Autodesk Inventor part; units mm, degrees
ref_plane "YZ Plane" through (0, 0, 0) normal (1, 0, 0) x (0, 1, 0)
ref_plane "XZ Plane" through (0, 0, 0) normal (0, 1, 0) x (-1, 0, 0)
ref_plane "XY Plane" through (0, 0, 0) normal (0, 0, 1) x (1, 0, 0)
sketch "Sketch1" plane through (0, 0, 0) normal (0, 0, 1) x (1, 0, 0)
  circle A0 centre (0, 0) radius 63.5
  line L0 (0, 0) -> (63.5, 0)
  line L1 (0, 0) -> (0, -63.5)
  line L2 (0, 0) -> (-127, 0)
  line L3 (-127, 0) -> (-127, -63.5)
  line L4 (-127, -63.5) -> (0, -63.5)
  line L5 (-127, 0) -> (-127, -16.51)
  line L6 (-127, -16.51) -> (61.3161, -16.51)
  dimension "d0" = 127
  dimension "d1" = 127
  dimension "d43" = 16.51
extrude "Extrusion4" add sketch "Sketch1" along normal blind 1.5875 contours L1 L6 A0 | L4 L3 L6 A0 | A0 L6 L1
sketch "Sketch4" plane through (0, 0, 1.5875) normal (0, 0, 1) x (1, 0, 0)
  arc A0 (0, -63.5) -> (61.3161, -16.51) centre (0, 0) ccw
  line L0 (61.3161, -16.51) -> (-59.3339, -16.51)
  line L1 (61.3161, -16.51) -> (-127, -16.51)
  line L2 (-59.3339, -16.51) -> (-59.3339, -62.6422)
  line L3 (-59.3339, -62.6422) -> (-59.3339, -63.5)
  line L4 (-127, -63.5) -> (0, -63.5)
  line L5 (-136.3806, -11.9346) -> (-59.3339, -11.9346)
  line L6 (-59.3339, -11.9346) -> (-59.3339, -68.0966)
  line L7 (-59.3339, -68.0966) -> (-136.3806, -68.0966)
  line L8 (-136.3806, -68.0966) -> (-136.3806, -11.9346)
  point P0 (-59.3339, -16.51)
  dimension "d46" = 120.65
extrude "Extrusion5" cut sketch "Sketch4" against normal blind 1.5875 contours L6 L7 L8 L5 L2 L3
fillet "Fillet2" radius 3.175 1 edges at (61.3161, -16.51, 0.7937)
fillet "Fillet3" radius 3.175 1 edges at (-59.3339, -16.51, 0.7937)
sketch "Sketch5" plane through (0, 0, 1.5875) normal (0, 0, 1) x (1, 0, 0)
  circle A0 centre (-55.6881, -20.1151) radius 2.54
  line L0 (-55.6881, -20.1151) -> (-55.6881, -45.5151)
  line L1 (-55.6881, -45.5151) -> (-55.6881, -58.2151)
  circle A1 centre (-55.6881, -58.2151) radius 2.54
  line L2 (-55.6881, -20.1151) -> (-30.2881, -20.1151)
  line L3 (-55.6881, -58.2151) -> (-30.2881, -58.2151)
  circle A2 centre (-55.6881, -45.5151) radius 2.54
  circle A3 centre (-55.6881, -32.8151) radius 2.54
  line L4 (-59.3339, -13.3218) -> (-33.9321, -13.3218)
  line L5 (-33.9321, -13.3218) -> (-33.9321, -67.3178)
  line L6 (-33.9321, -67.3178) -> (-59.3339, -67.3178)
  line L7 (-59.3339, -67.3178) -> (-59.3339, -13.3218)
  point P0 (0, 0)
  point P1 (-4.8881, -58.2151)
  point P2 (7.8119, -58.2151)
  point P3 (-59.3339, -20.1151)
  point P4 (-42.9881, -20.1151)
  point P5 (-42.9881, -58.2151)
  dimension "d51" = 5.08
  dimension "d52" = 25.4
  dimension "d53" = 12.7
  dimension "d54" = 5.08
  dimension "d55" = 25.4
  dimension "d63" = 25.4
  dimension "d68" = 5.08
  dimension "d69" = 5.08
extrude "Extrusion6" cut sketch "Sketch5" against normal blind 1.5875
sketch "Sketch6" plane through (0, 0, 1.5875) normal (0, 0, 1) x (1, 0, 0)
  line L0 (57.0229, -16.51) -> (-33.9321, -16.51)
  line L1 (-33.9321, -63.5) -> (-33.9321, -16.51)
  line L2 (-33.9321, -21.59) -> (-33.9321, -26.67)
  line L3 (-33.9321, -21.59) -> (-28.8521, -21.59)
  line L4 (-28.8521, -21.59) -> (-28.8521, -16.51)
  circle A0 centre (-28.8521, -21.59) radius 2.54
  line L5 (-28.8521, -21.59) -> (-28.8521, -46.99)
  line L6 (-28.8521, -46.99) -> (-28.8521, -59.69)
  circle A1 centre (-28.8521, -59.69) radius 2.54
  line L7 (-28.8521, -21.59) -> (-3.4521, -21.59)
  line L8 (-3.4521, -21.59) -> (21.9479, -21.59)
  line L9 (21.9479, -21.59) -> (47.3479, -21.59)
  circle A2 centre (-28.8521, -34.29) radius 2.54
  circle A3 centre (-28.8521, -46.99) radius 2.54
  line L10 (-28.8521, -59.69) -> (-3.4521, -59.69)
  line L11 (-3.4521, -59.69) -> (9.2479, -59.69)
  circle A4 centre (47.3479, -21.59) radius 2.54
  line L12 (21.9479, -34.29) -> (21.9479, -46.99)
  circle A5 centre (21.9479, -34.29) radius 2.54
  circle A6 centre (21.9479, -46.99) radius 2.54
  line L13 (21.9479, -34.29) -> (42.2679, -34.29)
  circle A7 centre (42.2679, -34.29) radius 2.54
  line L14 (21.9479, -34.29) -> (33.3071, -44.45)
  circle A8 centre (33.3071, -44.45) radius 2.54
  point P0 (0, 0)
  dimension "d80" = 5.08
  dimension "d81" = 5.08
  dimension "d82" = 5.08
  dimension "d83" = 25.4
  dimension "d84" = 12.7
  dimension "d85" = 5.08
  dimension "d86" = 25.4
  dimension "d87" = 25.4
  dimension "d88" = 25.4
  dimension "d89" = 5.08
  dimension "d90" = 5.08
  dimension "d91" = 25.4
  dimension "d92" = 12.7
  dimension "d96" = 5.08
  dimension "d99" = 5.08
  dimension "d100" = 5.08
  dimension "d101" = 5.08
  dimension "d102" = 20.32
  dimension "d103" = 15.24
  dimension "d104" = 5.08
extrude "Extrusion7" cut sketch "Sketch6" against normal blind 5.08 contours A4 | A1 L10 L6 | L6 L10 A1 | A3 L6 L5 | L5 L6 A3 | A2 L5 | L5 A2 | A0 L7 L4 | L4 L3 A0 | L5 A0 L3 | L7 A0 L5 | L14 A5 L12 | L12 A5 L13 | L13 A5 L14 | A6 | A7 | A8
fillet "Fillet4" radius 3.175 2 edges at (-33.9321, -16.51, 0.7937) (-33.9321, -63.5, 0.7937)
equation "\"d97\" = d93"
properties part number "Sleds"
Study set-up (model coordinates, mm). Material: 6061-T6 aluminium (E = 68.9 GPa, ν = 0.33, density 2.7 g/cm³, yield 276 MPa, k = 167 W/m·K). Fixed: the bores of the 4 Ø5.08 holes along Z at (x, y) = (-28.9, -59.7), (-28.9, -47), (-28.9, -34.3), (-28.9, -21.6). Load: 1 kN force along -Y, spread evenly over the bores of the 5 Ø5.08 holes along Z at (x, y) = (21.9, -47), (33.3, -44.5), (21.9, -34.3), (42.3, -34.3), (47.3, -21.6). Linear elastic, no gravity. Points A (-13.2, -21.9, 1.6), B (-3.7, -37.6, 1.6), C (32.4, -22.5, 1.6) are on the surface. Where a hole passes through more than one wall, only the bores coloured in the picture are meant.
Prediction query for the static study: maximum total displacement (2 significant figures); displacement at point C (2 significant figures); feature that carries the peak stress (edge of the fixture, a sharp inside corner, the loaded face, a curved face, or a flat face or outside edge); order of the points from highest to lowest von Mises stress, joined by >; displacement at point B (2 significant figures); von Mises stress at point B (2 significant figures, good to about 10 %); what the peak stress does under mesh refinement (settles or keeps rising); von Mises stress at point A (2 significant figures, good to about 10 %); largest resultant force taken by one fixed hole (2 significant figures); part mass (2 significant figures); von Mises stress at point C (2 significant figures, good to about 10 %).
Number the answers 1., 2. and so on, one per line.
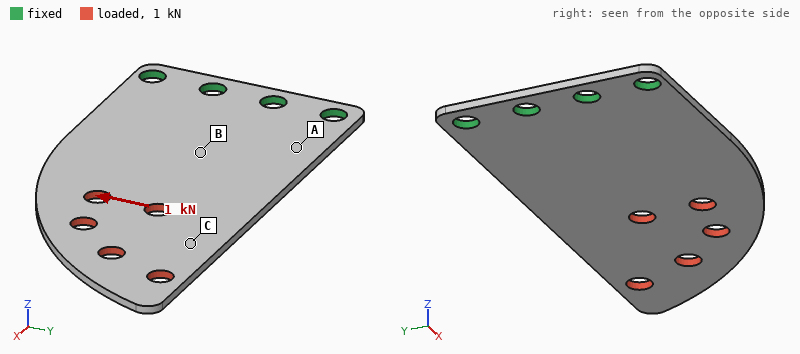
1. 0.19 mm
2. 0.12 mm
3. edge of the fixture
4. A > B > C
5. 0.030 mm
6. 34 MPa
7. keeps rising
8. 64 MPa
9. 1.5 kN
10. 15 g
11. 12 MPa
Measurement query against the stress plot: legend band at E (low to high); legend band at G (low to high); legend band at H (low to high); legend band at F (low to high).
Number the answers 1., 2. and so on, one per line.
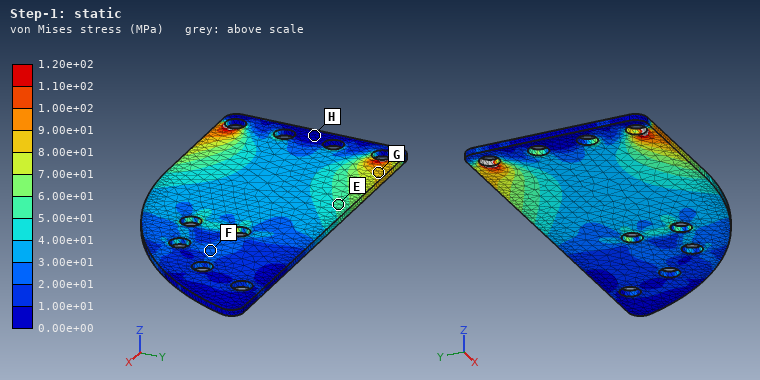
1. 5.00e+01 to 6.00e+01 MPa
2. 8.00e+01 to 9.00e+01 MPa
3. 0.00e+00 to 1.00e+01 MPa
4. 2.00e+01 to 3.00e+01 MPa
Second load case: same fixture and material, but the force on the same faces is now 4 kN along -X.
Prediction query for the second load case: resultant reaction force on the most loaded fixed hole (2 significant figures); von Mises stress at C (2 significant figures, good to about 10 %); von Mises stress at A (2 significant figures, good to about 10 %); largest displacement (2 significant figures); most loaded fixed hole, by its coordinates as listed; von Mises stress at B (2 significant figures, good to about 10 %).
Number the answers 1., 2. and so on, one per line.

1. 1.4 kN
2. 52 MPa
3. 72 MPa
4. 91 µm
5. (-28.9, -21.6)
6. 60 MPa
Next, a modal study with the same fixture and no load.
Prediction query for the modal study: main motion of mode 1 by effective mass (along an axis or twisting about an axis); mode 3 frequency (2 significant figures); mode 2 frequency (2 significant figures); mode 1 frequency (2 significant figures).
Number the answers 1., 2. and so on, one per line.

1. along Z
2. 1300 Hz
3. 950 Hz
4. 240 Hz
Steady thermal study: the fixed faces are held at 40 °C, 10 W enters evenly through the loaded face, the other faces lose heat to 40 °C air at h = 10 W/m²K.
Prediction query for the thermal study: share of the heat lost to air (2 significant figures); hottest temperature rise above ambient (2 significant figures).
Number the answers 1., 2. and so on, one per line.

1. 17 %
2. 50 K
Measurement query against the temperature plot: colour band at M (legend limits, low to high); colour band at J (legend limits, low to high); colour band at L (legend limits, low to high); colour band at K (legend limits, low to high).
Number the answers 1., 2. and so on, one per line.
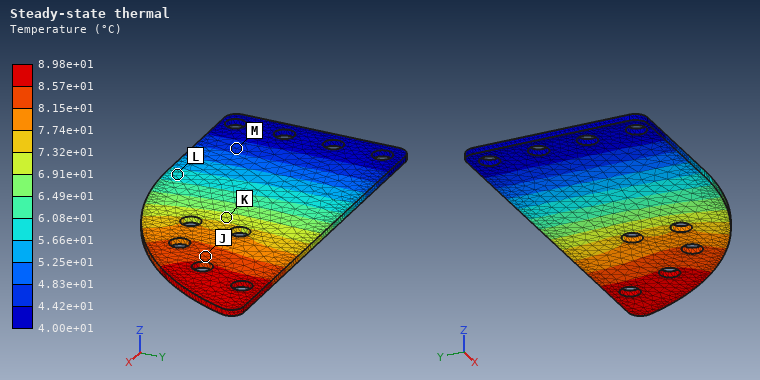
1. 4.42e+01 to 4.83e+01 °C
2. 8.15e+01 to 8.57e+01 °C
3. 5.66e+01 to 6.08e+01 °C
4. 6.91e+01 to 7.32e+01 °C
